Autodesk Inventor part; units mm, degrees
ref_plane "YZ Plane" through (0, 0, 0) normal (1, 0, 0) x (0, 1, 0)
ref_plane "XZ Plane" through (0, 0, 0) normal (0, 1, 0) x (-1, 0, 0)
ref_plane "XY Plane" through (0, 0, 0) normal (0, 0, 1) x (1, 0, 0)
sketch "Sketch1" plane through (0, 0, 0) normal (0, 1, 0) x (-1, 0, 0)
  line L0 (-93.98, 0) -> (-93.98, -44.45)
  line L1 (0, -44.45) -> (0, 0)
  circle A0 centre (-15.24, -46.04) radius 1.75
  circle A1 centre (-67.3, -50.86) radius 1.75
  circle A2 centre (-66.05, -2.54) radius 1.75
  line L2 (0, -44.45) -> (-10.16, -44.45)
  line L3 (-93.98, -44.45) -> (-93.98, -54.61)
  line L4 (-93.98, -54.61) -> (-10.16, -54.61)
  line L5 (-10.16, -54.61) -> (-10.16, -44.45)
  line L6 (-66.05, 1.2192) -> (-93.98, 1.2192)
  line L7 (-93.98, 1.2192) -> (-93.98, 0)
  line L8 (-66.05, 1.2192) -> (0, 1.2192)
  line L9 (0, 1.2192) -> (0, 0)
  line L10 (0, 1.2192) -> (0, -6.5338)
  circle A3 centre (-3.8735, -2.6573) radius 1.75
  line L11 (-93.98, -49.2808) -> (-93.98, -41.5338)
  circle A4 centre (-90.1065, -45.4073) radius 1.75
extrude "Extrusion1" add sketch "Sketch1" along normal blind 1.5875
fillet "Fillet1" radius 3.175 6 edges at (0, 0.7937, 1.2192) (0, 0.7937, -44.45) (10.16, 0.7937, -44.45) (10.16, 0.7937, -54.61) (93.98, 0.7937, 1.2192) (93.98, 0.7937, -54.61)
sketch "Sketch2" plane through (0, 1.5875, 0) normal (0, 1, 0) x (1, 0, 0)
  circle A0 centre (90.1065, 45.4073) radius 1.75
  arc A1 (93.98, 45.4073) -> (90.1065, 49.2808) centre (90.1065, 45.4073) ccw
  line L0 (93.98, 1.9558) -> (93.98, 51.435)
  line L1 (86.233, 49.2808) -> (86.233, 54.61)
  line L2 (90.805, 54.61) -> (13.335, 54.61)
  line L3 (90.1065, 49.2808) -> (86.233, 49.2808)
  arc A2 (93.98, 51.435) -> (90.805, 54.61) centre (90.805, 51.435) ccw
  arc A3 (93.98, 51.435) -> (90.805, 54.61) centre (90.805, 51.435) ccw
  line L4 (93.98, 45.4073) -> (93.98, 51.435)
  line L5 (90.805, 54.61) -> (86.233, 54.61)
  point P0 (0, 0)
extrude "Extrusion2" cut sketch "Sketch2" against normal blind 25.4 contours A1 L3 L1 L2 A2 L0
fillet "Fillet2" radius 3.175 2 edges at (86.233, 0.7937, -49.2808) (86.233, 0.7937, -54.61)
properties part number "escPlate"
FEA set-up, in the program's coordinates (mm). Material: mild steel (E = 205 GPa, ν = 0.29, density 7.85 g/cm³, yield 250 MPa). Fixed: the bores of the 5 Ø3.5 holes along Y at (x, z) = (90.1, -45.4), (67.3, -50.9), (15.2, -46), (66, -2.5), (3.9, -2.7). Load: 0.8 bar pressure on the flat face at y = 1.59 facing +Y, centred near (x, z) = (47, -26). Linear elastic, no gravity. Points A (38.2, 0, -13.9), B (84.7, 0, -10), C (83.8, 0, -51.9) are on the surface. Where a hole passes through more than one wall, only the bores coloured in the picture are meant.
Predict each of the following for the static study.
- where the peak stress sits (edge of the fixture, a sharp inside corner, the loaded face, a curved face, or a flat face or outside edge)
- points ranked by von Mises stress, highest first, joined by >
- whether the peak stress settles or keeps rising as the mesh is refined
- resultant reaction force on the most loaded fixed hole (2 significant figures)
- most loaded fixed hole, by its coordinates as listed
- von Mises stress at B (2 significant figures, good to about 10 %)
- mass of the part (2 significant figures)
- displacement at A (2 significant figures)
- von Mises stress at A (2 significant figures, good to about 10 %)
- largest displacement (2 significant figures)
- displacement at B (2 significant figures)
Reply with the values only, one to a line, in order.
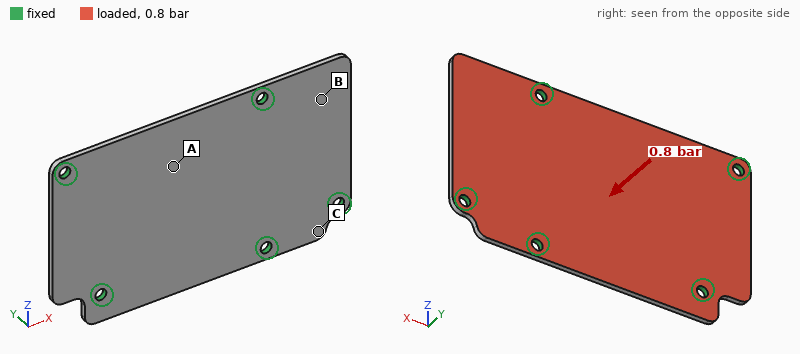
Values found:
edge of the fixture
A > B > C
keeps rising
120 N
(66, -2.5)
16 MPa
63 g
51 µm
26 MPa
51 µm
29 µm
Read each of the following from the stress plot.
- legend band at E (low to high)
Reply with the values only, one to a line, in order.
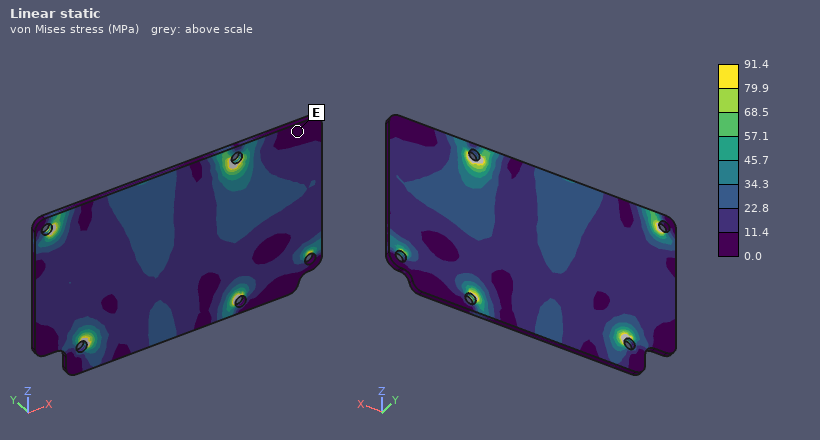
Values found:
0.0 to 11.4 MPa
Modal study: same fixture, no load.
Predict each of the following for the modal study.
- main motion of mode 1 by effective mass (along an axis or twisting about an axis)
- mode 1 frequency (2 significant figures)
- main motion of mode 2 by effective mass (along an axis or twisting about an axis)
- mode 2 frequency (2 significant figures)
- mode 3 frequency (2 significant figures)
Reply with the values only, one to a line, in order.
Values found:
along Y
2100 Hz
along Y
2300 Hz
3200 Hz
